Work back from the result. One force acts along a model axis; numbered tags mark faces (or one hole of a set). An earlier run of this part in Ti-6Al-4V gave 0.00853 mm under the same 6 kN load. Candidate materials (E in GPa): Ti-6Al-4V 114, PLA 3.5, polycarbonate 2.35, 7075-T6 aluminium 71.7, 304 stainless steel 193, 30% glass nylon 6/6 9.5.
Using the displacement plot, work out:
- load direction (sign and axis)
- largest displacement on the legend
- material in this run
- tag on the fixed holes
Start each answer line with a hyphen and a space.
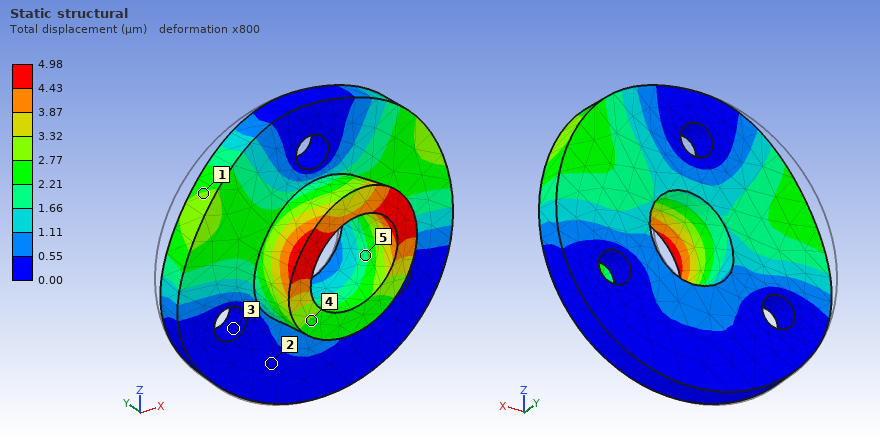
- +X
- 4.98 µm
- 304 stainless steel
- 3
